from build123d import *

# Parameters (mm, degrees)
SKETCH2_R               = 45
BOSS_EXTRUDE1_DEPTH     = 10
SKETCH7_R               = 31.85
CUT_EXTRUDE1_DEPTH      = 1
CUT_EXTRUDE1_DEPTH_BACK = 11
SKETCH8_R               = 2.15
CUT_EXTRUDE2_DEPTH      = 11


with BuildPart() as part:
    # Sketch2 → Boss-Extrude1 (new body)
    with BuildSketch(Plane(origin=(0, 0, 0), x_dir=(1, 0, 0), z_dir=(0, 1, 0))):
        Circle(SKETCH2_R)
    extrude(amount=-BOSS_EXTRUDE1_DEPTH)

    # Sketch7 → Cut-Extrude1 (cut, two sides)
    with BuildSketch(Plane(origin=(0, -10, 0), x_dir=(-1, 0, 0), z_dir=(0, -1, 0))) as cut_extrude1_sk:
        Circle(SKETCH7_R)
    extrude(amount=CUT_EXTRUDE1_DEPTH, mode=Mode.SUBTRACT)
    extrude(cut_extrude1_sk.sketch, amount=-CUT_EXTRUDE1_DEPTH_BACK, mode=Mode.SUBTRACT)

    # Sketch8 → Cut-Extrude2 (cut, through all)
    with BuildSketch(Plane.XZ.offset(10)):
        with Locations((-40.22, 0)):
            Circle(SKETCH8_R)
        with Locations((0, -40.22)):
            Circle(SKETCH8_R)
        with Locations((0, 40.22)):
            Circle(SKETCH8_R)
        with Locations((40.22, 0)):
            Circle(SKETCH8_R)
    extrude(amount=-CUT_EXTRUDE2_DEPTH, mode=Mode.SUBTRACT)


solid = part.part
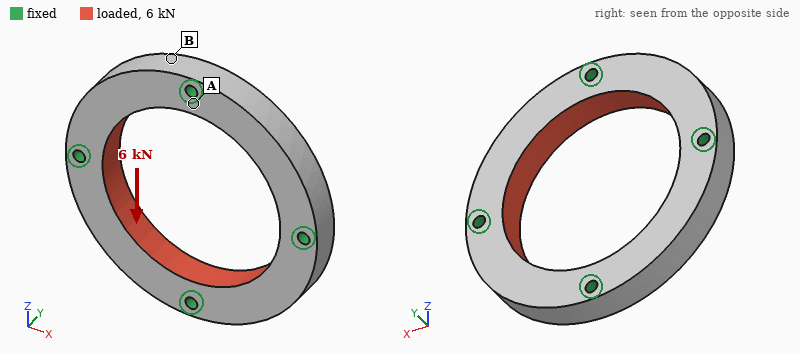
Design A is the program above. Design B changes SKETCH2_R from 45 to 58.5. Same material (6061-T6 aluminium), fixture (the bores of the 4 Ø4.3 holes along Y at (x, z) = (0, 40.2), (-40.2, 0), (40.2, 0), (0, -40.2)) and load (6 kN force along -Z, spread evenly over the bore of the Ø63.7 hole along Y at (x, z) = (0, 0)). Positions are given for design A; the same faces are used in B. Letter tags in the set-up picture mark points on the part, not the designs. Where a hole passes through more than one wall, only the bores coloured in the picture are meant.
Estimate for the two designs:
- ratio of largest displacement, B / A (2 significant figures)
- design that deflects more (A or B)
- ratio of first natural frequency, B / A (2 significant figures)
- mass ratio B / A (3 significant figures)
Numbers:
0.51
A
0.55
2.41
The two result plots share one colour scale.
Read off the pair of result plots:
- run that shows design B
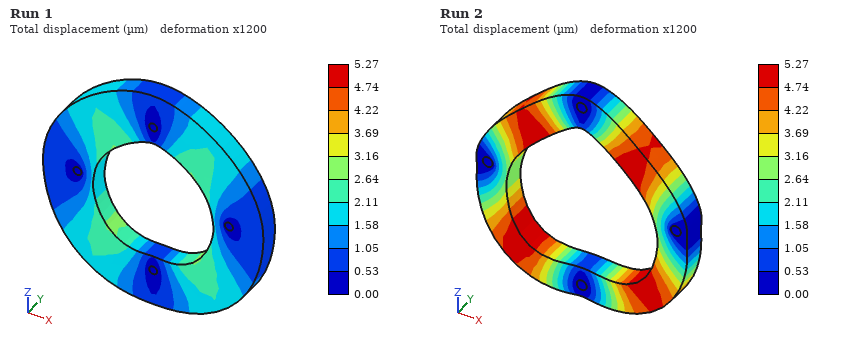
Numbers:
Run 1
